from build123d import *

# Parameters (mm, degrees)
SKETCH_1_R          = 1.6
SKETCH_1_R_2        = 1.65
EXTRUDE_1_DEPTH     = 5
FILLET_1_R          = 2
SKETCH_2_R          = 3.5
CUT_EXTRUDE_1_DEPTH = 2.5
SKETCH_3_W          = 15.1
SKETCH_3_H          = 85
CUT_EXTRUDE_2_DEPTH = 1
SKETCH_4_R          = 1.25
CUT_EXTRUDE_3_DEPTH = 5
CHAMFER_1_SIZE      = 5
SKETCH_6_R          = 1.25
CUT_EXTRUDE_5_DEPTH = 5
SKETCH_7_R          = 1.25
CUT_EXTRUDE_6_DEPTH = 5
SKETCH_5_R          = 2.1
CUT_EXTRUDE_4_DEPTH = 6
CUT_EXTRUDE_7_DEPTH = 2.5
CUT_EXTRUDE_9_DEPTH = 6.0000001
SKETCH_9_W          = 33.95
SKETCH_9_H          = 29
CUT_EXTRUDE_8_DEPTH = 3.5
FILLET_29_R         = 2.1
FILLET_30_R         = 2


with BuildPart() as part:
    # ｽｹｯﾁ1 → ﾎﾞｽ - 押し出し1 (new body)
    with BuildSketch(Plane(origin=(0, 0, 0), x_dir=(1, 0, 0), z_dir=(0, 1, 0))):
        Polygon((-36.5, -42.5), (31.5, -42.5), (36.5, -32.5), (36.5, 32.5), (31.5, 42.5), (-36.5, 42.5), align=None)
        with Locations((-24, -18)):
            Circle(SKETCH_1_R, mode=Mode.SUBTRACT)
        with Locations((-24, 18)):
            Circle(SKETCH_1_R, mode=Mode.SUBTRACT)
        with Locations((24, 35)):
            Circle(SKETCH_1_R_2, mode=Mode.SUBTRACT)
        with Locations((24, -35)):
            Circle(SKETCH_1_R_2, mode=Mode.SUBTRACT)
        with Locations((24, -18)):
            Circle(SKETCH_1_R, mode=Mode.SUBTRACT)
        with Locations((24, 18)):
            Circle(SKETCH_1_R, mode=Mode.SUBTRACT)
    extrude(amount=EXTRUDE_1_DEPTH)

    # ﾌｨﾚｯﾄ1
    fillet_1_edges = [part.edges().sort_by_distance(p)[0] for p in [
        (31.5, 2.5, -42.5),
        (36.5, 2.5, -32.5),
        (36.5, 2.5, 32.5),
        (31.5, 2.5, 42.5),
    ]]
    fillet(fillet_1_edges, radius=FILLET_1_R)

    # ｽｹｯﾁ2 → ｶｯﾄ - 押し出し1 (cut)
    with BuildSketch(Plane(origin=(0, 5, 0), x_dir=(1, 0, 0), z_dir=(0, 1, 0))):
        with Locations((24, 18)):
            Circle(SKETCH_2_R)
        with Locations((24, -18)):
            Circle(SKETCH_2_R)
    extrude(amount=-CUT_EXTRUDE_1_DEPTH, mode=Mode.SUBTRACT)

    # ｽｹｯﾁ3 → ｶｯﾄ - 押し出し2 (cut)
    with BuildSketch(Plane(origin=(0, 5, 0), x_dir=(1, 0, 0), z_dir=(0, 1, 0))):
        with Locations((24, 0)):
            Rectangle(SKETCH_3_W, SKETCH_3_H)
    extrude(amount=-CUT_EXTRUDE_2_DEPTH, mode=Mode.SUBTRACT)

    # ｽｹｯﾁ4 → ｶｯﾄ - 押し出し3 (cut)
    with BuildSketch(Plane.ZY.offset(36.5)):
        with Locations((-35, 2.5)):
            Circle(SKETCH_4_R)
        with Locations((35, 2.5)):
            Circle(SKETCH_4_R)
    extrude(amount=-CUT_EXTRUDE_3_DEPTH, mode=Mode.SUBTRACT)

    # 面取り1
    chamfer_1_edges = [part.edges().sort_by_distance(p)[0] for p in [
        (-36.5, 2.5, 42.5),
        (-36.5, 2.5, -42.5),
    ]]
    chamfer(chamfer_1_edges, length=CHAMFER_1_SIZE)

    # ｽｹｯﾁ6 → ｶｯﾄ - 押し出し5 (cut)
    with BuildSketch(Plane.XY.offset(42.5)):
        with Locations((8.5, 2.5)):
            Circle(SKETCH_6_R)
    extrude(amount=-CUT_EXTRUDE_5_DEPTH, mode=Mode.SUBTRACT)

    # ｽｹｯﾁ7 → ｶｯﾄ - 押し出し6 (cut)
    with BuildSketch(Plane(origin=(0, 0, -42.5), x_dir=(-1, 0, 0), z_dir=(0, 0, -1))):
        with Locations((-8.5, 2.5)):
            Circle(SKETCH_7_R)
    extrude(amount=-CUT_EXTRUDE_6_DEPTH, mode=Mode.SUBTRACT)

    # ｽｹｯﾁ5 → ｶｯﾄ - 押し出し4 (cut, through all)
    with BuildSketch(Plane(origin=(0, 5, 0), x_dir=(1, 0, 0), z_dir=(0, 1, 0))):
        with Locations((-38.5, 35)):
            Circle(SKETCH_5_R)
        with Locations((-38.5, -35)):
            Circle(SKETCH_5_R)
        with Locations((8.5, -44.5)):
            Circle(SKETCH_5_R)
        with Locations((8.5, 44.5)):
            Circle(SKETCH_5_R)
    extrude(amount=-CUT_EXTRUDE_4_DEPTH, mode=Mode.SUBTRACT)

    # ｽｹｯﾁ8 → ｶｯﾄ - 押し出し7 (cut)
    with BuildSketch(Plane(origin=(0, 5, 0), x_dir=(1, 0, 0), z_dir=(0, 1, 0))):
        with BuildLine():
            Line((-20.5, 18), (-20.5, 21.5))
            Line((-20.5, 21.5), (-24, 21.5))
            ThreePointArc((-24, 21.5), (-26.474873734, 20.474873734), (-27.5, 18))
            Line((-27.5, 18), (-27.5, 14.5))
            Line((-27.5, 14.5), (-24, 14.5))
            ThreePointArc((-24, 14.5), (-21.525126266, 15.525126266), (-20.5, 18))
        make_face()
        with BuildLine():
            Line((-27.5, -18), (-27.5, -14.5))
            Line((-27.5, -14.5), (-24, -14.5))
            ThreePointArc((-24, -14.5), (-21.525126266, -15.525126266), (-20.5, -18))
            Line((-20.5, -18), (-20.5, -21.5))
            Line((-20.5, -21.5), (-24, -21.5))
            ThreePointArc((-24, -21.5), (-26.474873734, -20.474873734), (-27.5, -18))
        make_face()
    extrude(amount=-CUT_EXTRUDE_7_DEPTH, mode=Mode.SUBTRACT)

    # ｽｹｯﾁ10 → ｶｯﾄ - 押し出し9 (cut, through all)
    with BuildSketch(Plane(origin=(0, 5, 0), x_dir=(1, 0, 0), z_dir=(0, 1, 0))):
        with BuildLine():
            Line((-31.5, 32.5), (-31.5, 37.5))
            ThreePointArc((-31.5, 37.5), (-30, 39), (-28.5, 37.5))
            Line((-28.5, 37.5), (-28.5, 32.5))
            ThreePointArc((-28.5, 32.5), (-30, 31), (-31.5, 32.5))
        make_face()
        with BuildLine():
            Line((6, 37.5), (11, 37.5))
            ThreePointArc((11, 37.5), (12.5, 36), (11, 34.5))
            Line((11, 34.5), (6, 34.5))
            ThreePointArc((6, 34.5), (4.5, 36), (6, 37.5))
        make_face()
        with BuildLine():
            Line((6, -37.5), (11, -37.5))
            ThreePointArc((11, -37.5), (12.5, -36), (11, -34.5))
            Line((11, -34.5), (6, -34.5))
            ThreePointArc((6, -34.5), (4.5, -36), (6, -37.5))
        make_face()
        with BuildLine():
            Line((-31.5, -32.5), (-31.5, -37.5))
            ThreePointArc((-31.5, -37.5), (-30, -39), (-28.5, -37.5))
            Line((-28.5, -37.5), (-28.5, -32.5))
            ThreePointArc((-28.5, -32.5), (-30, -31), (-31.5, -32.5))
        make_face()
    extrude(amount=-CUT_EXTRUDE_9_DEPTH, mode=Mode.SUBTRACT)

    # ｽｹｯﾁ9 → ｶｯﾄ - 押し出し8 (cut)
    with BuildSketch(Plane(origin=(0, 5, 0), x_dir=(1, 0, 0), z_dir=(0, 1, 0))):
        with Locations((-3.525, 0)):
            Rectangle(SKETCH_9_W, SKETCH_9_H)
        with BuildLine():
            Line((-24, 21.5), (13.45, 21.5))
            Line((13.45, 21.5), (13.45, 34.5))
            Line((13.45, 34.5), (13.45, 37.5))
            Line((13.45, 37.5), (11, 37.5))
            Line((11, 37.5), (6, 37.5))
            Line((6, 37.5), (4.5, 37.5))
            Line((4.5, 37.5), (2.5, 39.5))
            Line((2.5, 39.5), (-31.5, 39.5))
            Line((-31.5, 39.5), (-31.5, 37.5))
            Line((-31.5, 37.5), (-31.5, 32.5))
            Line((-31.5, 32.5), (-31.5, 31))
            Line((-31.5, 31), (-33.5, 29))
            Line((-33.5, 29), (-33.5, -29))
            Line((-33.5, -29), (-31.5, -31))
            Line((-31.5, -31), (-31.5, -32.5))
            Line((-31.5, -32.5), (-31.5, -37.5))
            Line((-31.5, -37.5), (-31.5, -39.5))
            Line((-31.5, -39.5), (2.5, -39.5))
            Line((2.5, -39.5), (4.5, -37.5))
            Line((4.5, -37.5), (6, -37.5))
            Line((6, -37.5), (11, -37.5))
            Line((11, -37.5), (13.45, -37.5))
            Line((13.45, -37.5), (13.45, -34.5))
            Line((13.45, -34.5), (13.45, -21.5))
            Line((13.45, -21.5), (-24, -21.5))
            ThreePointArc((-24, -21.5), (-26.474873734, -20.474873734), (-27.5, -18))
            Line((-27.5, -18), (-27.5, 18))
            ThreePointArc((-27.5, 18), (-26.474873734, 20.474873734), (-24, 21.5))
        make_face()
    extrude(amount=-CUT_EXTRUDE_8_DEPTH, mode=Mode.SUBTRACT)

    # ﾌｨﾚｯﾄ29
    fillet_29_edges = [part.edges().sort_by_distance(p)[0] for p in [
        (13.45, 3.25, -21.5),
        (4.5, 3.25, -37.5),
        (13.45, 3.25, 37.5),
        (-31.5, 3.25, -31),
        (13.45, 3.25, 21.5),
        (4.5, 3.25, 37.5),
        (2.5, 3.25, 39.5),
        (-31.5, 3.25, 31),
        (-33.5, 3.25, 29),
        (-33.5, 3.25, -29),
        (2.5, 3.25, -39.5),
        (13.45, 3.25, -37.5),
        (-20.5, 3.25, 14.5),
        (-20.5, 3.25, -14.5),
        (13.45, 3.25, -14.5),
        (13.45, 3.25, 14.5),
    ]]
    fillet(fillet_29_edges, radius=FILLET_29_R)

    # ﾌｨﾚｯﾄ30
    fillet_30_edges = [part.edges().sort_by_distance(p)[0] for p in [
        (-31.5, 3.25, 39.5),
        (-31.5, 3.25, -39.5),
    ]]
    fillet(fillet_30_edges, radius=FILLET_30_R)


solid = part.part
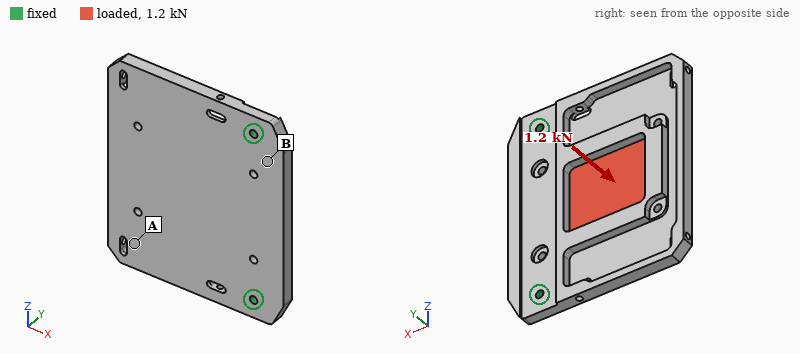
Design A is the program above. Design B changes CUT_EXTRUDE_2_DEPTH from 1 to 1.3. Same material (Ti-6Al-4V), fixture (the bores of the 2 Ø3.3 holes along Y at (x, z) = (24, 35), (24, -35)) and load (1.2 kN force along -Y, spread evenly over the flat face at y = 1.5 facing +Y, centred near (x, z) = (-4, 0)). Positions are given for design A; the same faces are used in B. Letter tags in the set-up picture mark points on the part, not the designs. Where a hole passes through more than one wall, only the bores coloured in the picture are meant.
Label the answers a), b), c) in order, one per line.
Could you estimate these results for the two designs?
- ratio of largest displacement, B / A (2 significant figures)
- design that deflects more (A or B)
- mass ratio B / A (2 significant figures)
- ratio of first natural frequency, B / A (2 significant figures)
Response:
a) 1.1
b) B
c) 0.98
d) 0.94
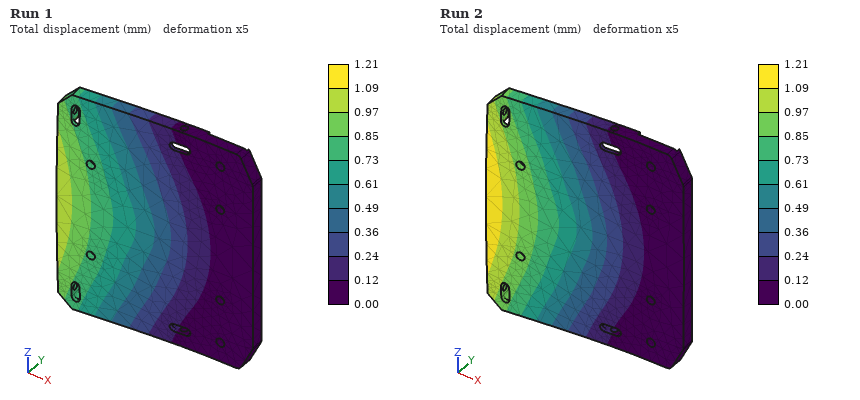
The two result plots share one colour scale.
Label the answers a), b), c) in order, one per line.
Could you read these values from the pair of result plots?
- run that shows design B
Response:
a) Run 2
